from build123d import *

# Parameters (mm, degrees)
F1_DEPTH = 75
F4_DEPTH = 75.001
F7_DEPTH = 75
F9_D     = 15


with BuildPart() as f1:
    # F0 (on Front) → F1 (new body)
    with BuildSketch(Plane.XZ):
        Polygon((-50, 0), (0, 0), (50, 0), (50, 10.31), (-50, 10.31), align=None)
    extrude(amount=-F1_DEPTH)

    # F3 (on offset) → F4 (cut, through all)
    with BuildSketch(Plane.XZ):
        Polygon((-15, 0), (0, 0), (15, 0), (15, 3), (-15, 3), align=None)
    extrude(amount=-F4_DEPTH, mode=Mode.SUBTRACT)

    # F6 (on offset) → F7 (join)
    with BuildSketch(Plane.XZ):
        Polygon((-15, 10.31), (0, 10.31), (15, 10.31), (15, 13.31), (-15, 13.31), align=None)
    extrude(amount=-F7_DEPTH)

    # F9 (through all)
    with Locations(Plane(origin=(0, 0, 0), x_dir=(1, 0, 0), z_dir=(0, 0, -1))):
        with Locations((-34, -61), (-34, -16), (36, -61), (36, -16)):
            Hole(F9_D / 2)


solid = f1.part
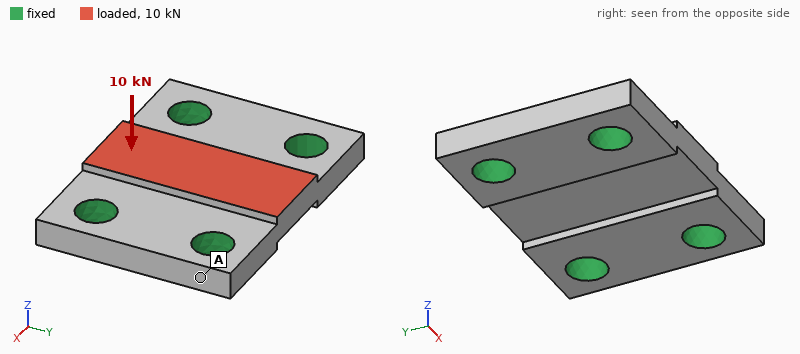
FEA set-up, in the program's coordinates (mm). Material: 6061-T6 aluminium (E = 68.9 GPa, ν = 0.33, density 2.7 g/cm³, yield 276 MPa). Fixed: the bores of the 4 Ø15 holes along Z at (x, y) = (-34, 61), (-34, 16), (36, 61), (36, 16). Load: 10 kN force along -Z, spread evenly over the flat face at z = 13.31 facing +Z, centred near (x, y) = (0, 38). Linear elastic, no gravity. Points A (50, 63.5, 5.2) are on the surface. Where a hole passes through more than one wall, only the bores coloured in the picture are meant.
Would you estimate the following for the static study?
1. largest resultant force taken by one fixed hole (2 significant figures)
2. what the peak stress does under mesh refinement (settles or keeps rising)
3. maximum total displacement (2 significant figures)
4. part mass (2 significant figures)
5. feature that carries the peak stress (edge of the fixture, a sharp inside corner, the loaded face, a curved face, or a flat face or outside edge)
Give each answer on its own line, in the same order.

3.4 kN
keeps rising
26 µm
190 g
edge of the fixture
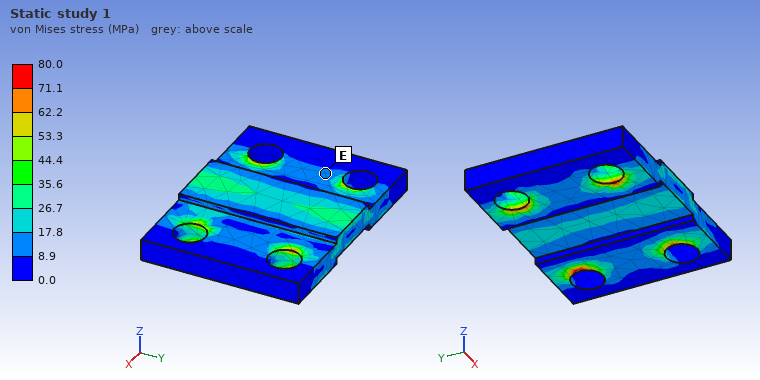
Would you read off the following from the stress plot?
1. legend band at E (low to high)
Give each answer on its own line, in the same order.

8.9 to 17.8 MPa
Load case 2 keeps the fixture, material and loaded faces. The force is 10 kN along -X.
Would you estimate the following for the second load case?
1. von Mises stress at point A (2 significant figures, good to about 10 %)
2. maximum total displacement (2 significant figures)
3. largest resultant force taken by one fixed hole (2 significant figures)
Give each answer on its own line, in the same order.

1.6 MPa
5.3 µm
2.8 kN
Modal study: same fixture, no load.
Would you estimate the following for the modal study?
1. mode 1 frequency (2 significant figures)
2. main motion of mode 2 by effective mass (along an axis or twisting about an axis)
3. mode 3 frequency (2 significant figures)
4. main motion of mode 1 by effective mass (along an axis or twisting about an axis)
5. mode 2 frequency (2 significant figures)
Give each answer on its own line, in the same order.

12 kHz
twisting about X
18 kHz
along Z
14 kHz
